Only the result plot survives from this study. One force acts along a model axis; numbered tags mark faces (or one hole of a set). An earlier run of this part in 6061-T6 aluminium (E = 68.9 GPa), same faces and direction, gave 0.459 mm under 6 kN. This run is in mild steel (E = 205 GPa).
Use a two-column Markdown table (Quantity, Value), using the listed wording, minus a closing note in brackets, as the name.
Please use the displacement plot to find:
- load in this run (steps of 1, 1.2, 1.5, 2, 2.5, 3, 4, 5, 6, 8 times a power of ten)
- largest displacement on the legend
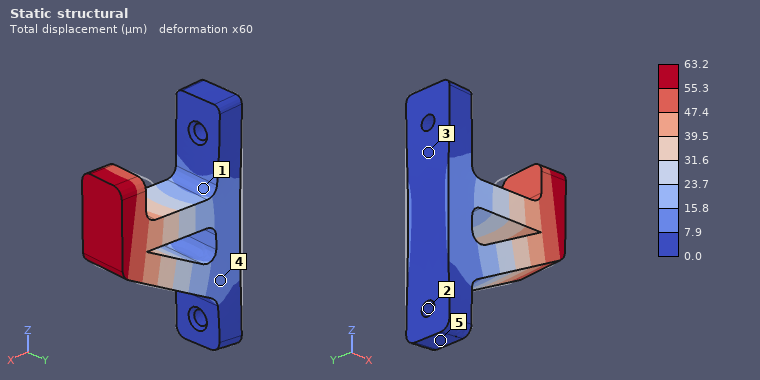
| Quantity | Value |
|---|---|
| load in this run | 2.5 kN |
| largest displacement on the legend | 63.2 µm |
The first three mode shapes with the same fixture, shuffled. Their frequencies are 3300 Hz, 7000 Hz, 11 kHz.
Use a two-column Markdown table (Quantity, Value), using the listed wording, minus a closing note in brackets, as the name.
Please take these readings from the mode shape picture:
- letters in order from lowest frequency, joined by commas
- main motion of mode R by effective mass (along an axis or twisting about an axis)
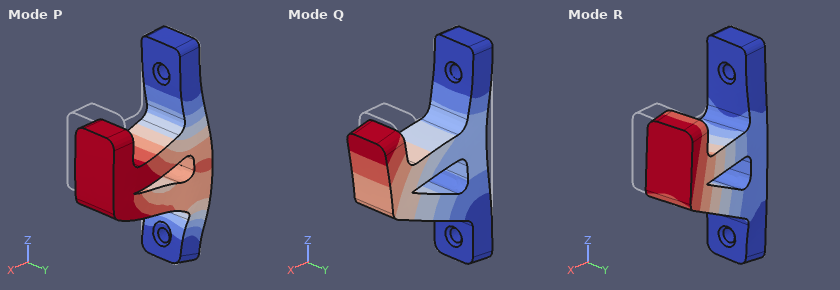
| Quantity | Value |
|---|---|
| letters in order from lowest frequency, joined by commas | R, Q, P |
| main motion of mode R by effective mass | along Y |
